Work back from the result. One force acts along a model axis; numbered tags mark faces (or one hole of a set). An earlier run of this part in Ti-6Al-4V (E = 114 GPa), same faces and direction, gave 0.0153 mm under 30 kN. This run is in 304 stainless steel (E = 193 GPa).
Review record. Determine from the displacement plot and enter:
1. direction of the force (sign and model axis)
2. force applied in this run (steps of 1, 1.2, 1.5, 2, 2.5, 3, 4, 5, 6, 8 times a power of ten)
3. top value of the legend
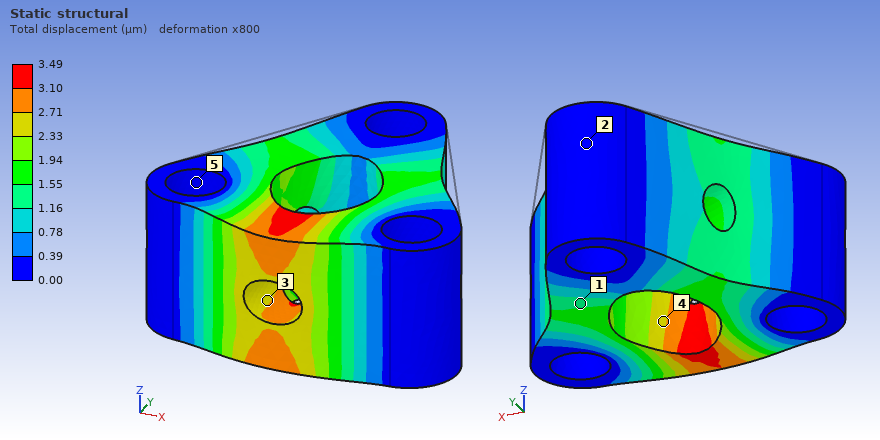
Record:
-Y
12 kN
3.49 µm
